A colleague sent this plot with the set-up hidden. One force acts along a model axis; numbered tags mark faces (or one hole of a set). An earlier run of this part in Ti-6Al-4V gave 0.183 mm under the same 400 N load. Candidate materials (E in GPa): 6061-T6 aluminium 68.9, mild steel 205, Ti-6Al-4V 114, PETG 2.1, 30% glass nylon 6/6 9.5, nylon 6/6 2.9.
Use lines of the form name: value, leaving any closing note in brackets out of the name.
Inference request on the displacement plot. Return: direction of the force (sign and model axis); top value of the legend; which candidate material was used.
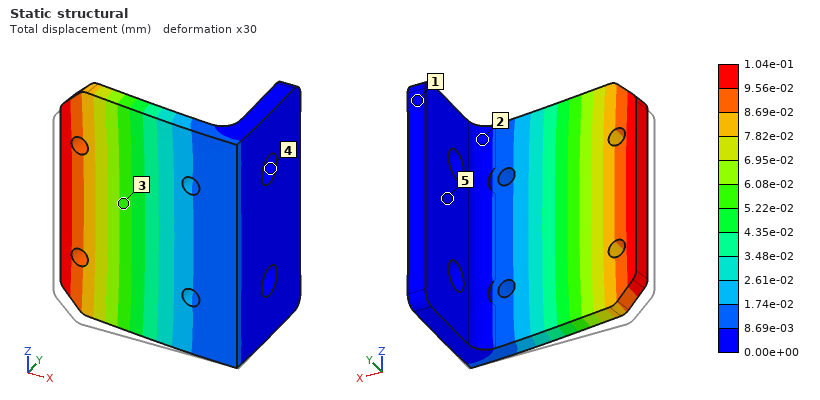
direction of the force: +Y
top value of the legend: 1.04e-01 mm
which candidate material was used: mild steel
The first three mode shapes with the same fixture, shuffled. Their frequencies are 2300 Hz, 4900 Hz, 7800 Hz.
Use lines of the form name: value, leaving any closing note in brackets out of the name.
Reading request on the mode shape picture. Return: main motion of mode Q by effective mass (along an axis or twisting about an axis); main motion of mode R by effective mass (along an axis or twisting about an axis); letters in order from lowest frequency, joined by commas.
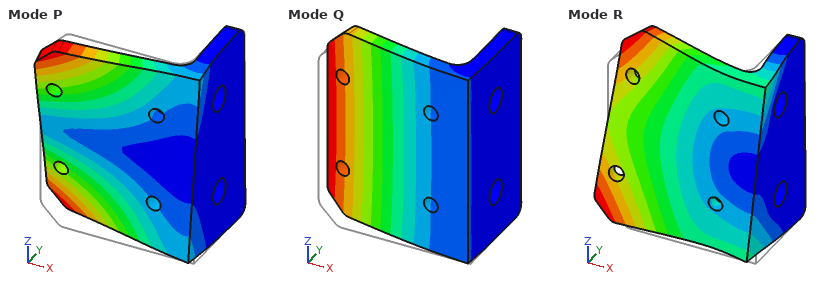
main motion of mode Q by effective mass: along Y
main motion of mode R by effective mass: along Z
letters in order from lowest frequency, joined by commas: Q, P, R
